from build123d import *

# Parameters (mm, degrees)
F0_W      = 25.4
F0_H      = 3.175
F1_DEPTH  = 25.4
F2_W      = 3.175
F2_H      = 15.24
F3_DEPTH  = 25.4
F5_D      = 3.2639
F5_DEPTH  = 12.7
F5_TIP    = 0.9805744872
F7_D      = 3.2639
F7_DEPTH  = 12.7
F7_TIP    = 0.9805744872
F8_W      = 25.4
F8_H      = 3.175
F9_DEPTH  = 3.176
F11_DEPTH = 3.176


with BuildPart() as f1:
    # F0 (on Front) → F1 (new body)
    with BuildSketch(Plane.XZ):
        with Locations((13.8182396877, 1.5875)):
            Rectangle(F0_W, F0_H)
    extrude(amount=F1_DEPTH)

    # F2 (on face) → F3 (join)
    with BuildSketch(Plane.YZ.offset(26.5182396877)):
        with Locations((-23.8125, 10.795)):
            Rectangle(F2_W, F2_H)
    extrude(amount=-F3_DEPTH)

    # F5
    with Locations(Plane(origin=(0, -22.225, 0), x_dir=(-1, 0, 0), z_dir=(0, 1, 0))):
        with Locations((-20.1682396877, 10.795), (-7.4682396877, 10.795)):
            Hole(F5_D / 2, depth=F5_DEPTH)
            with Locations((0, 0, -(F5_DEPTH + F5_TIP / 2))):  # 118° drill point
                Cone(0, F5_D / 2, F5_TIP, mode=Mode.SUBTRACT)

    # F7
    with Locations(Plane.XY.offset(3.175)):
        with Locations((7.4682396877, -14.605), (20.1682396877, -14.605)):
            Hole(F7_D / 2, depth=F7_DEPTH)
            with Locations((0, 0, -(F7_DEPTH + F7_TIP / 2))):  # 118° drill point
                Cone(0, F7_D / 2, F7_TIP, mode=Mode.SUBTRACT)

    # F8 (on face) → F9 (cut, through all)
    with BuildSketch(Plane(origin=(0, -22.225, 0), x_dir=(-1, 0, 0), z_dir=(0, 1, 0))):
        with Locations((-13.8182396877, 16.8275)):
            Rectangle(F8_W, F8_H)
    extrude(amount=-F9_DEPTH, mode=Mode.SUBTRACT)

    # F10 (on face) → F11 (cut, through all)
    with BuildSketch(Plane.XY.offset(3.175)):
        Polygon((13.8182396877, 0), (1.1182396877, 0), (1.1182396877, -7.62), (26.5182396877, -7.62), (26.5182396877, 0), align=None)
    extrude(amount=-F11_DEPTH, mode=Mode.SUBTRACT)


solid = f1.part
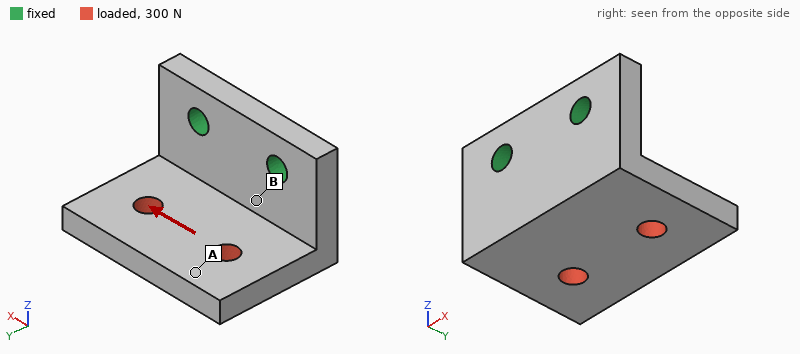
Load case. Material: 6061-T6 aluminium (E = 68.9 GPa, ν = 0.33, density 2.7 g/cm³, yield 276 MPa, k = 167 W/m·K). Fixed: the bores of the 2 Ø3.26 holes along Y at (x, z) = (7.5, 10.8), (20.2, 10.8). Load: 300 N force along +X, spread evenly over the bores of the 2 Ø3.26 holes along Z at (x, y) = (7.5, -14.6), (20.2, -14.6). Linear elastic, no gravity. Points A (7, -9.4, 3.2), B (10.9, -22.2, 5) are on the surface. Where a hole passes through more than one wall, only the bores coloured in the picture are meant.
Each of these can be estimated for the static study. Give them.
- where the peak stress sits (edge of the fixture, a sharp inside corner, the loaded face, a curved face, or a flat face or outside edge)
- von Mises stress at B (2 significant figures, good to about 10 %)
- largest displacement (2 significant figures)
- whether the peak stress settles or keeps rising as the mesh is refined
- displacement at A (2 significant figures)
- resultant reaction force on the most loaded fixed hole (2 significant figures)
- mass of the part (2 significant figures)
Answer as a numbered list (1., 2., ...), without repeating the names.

1. edge of the fixture
2. 32 MPa
3. 30 µm
4. keeps rising
5. 24 µm
6. 280 N
7. 6.2 g
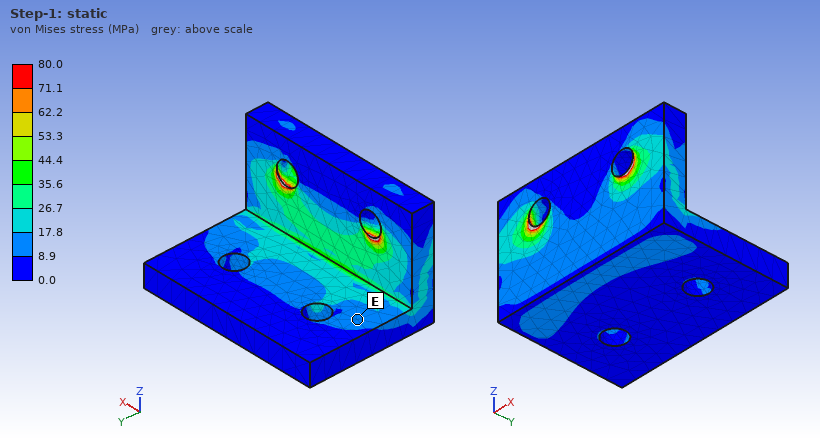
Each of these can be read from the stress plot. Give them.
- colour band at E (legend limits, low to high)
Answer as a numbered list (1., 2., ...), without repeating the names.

1. 8.9 to 17.8 MPa
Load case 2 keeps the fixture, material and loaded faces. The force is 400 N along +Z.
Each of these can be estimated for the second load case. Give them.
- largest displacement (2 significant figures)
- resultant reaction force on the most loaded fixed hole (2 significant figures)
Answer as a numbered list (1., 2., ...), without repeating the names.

1. 0.15 mm
2. 200 N
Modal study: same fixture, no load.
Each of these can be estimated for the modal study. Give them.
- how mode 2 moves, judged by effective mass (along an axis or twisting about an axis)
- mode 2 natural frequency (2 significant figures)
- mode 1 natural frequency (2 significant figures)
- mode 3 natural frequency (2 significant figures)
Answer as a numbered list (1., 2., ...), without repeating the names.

1. along X
2. 9700 Hz
3. 5500 Hz
4. 15 kHz
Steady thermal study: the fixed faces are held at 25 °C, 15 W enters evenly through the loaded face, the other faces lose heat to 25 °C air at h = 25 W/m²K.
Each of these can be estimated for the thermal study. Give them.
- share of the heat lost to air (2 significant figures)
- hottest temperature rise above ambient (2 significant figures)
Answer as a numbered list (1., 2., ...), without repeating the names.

1. 3.1 %
2. 21 K
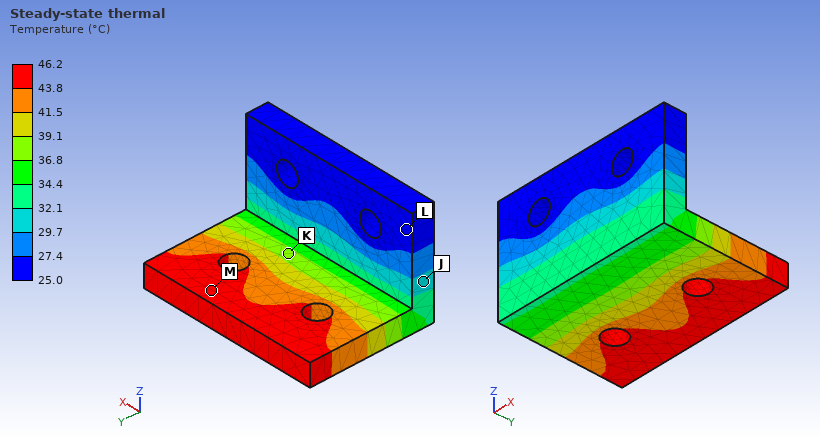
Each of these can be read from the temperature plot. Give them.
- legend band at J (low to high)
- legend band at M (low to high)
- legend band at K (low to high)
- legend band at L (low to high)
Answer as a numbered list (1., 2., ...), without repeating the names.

1. 29.7 to 32.1 °C
2. 43.8 to 46.2 °C
3. 36.8 to 39.1 °C
4. 25.0 to 27.4 °C
